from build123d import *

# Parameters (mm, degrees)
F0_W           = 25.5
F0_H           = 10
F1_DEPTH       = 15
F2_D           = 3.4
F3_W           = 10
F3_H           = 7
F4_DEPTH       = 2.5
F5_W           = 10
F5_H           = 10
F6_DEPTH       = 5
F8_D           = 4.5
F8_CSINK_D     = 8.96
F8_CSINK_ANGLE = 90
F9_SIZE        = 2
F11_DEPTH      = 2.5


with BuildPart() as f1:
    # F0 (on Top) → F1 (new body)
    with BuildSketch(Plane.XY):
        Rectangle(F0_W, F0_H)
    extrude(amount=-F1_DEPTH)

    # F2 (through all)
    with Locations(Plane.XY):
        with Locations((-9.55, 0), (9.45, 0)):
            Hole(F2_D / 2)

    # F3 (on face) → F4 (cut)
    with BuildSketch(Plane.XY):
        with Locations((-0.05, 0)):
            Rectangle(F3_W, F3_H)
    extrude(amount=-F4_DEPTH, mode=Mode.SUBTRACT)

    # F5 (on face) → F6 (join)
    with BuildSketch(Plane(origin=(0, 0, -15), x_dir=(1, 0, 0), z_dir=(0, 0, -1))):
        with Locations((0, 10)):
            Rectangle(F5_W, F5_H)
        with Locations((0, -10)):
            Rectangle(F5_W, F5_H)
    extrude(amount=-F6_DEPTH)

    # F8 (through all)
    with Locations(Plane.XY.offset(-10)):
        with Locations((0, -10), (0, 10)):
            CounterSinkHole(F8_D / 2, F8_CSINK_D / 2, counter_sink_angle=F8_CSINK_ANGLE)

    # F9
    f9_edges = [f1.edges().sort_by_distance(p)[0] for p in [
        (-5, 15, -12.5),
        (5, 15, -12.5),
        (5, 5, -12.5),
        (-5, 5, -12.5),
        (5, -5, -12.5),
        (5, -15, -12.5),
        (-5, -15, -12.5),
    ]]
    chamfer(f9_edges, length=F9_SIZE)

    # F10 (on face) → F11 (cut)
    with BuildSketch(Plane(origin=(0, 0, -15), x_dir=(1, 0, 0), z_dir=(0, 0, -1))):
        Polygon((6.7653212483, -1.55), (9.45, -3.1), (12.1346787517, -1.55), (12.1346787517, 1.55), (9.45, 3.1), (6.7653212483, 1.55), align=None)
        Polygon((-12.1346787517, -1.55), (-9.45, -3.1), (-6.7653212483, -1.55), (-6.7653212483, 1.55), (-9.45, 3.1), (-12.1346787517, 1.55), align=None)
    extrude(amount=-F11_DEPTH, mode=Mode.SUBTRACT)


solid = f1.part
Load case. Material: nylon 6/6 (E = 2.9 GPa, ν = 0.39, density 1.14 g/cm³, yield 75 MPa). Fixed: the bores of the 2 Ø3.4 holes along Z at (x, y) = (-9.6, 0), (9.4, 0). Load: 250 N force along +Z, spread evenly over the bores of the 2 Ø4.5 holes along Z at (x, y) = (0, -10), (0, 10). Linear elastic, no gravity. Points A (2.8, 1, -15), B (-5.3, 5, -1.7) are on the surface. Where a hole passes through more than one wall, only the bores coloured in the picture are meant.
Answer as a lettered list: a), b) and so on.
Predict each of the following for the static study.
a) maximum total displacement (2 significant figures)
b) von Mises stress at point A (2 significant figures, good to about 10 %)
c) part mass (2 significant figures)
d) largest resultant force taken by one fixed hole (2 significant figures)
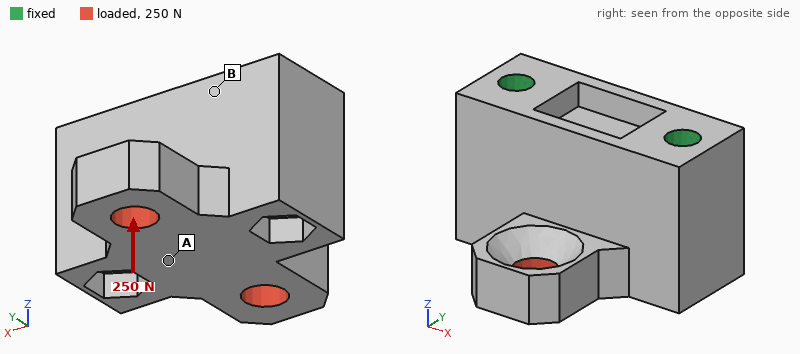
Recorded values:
a) 0.16 mm
b) 8.0 MPa
c) 4.6 g
d) 140 N
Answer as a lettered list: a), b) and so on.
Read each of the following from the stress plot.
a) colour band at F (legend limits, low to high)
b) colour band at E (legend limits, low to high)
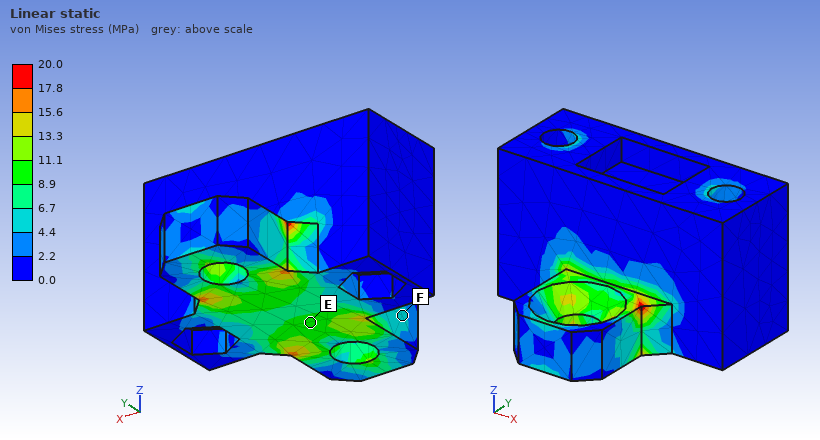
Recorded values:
a) 4.4 to 6.7 MPa
b) 8.9 to 11.1 MPa
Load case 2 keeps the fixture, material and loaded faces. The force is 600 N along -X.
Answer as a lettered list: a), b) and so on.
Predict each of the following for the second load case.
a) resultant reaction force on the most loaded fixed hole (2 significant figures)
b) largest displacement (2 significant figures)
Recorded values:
a) 340 N
b) 0.16 mm
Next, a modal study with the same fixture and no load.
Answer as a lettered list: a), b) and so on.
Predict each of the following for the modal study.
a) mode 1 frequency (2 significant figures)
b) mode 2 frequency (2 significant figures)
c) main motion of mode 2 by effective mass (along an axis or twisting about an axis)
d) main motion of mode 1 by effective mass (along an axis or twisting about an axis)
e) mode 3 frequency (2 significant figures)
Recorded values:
a) 7200 Hz
b) 8400 Hz
c) along Z
d) twisting about X
e) 11 kHz
